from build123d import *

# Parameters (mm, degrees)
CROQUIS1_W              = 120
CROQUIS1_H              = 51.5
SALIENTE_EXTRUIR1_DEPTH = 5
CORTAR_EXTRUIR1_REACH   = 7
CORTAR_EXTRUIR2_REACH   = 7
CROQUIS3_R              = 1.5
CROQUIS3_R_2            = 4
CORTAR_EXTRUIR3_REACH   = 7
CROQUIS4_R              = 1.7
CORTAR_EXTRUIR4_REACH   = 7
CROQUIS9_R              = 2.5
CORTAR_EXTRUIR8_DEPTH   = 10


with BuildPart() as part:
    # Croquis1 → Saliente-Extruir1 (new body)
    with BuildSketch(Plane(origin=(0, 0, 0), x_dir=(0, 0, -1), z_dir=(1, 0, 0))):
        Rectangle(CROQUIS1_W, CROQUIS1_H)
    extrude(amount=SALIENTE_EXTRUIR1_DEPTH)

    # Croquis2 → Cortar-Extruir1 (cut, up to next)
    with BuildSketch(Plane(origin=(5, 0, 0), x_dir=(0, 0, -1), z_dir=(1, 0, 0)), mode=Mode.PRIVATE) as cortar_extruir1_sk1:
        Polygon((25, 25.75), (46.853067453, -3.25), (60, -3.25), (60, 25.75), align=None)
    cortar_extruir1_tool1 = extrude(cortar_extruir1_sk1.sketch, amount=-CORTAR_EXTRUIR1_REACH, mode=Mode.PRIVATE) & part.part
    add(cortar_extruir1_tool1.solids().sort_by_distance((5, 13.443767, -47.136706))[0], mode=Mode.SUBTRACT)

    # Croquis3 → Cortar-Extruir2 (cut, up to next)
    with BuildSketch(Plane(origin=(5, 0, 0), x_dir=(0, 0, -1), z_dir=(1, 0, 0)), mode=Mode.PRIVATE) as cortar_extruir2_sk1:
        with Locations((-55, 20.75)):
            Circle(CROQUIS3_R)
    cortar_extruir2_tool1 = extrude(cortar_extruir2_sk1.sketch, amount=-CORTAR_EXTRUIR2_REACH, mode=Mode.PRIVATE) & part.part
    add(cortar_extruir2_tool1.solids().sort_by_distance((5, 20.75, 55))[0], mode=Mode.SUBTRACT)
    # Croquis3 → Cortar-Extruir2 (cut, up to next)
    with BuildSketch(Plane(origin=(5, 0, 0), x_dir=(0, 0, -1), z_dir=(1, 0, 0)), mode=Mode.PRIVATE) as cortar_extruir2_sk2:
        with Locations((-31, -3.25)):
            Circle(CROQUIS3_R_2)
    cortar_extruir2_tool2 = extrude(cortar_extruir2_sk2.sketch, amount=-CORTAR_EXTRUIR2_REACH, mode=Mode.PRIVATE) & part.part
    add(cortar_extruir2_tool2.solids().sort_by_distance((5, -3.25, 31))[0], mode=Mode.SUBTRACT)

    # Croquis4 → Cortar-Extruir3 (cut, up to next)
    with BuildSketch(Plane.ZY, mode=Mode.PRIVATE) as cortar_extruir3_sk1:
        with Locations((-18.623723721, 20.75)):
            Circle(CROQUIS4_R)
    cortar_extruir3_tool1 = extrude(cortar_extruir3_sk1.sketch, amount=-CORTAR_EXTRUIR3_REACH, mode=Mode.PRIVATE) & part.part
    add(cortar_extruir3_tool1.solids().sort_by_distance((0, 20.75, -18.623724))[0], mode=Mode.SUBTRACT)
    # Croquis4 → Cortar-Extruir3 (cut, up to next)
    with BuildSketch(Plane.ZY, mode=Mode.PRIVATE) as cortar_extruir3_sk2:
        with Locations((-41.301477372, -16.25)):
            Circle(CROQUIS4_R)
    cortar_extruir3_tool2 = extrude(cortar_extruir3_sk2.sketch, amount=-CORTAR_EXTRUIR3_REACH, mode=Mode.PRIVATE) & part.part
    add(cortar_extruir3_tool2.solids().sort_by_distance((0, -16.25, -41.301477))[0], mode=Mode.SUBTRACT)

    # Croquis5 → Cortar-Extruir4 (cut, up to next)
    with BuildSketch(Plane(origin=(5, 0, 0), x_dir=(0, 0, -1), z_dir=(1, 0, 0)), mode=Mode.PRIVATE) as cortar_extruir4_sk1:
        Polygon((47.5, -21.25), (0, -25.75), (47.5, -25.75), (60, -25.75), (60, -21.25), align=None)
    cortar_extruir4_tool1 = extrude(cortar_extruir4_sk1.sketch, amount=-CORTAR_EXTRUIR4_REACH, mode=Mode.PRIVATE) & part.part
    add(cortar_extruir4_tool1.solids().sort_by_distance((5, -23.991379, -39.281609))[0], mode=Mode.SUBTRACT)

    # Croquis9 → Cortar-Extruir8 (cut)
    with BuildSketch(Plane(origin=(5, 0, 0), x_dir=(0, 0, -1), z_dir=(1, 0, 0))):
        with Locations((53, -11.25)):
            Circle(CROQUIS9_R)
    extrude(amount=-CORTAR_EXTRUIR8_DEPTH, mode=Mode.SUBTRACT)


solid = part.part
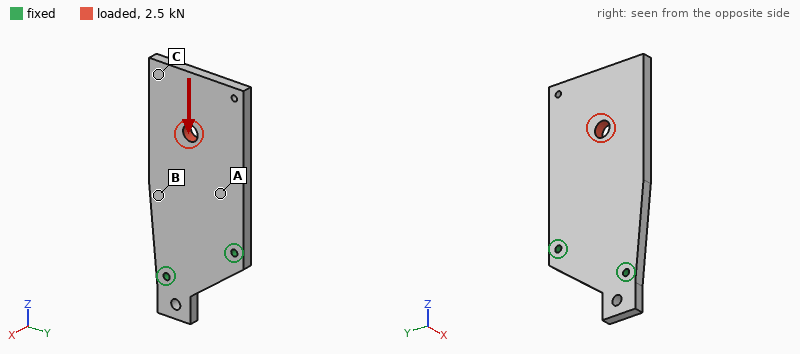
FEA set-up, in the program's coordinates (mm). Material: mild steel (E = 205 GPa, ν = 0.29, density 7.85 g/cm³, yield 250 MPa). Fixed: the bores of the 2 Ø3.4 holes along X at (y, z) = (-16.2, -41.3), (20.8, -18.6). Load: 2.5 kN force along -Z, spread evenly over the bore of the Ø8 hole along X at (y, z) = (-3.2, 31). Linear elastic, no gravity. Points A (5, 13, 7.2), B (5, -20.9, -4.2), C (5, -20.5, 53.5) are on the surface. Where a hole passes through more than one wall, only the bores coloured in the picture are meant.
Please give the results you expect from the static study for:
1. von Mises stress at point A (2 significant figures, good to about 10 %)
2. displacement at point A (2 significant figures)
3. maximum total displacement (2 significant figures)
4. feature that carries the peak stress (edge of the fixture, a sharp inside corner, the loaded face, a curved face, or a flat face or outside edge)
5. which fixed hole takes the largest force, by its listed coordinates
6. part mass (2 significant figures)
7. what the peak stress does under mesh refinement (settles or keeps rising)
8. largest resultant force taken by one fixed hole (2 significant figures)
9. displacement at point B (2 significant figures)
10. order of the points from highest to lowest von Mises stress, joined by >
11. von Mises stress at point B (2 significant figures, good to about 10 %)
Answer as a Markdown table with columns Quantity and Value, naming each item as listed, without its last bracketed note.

| Quantity | Value |
|---|---|
| von Mises stress at point A | 8.0 MPa |
| displacement at point A | 2.5 µm |
| maximum total displacement | 8.9 µm |
| feature that carries the peak stress | edge of the fixture |
| which fixed hole takes the largest force, by its listed coordinates | (-16.2, -41.3) |
| part mass | 210 g |
| what the peak stress does under mesh refinement | keeps rising |
| largest resultant force taken by one fixed hole | 1.6 kN |
| displacement at point B | 4.0 µm |
| order of the points from highest to lowest von Mises stress, joined by > | B > A > C |
| von Mises stress at point B | 14 MPa |
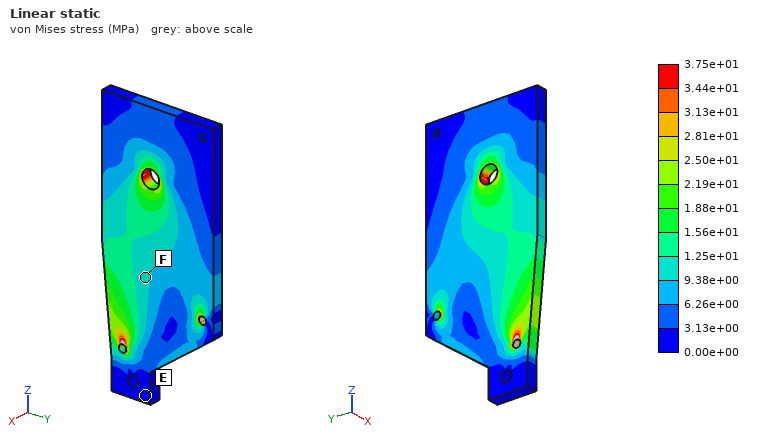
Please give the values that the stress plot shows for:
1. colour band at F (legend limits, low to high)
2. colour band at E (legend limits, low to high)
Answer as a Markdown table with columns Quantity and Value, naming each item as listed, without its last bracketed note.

| Quantity | Value |
|---|---|
| colour band at F | 9.38e+00 to 1.25e+01 MPa |
| colour band at E | 0.00e+00 to 3.13e+00 MPa |
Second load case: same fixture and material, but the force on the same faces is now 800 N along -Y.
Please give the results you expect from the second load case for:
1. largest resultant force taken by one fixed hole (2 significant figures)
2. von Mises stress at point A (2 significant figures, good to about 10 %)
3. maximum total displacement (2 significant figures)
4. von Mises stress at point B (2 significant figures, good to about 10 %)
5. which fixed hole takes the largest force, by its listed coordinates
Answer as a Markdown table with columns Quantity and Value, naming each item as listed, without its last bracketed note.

| Quantity | Value |
|---|---|
| largest resultant force taken by one fixed hole | 1.3 kN |
| von Mises stress at point A | 8.1 MPa |
| maximum total displacement | 13 µm |
| von Mises stress at point B | 10 MPa |
| which fixed hole takes the largest force, by its listed coordinates | (20.8, -18.6) |
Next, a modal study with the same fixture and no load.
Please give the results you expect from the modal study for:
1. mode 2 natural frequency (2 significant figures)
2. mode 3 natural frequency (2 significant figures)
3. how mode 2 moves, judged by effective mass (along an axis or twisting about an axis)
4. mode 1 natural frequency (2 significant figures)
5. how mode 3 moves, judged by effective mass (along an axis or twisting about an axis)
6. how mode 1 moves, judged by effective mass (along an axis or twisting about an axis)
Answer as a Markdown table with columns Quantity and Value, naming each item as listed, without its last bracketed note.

| Quantity | Value |
|---|---|
| mode 2 natural frequency | 1800 Hz |
| mode 3 natural frequency | 3200 Hz |
| how mode 2 moves, judged by effective mass | twisting about Z |
| mode 1 natural frequency | 530 Hz |
| how mode 3 moves, judged by effective mass | along X |
| how mode 1 moves, judged by effective mass | along X |
